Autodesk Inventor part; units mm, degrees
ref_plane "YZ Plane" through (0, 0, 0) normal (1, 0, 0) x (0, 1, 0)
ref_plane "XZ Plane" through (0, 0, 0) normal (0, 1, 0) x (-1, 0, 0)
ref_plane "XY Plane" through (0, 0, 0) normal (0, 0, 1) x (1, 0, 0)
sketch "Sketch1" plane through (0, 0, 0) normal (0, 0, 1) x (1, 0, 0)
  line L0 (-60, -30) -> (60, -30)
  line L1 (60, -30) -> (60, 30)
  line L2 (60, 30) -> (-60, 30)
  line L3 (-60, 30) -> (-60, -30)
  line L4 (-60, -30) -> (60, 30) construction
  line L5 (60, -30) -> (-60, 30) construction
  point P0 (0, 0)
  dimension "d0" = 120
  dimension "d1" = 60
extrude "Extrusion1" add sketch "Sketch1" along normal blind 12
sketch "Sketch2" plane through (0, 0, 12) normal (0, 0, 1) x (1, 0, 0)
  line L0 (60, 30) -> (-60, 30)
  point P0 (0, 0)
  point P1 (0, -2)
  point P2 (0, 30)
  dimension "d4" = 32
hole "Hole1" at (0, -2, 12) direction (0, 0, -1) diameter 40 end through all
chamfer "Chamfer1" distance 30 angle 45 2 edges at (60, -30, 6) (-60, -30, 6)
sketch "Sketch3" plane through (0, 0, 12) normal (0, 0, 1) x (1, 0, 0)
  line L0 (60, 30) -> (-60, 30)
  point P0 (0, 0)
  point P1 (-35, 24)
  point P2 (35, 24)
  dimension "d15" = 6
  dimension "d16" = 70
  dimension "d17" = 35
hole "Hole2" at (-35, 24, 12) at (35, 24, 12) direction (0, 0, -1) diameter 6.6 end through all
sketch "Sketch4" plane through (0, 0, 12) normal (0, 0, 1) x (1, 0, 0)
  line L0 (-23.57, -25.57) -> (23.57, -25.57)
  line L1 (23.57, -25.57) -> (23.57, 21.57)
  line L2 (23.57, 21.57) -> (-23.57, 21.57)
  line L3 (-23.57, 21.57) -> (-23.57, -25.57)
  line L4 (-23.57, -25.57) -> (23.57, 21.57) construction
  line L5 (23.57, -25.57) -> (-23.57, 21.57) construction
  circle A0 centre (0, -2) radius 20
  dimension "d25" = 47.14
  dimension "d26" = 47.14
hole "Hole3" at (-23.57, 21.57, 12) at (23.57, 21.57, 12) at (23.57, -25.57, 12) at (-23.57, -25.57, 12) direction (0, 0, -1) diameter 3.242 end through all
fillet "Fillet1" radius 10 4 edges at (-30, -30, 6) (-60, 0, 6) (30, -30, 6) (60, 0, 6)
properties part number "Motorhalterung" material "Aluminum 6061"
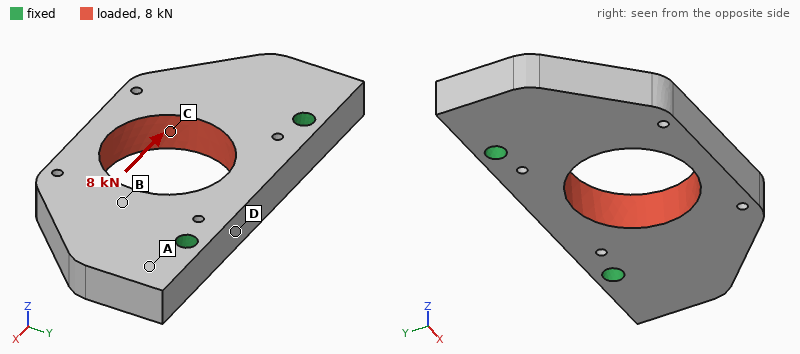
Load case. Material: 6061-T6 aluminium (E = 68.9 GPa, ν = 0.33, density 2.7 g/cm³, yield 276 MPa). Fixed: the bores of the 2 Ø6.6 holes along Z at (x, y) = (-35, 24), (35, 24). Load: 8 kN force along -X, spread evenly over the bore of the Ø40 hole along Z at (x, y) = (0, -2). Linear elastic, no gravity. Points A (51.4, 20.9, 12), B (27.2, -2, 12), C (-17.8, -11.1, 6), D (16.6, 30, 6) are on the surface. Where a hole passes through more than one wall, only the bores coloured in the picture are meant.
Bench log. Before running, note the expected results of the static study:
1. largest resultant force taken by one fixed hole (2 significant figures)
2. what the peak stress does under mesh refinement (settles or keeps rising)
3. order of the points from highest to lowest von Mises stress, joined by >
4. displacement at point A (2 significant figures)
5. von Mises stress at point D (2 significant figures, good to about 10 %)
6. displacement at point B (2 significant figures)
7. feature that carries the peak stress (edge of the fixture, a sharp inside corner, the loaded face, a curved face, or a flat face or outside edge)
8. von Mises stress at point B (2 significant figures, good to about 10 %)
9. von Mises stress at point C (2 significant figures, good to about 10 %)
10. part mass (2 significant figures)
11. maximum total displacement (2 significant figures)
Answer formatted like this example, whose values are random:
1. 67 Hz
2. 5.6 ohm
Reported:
1. 4.5 kN
2. keeps rising
3. D > C > B > A
4. 16 µm
5. 37 MPa
6. 26 µm
7. edge of the fixture
8. 17 MPa
9. 27 MPa
10. 160 g
11. 49 µm
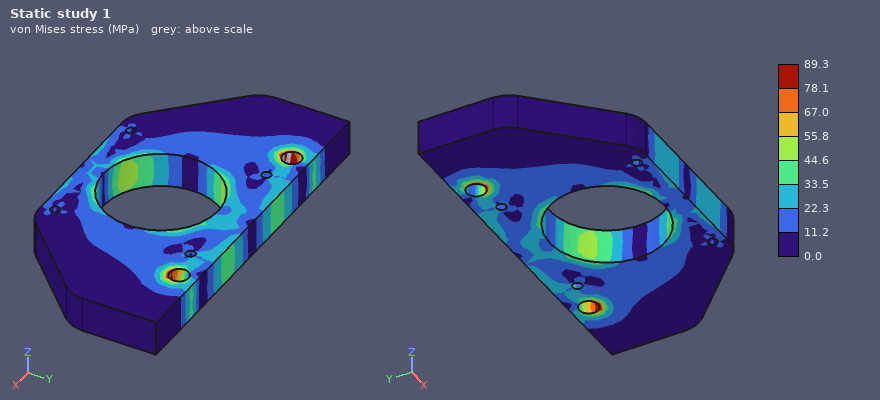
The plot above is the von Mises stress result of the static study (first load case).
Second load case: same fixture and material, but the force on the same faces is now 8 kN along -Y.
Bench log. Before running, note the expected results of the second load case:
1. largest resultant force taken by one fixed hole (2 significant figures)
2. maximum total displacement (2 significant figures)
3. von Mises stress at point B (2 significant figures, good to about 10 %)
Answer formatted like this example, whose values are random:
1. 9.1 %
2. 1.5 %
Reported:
1. 4.1 kN
2. 18 µm
3. 15 MPa
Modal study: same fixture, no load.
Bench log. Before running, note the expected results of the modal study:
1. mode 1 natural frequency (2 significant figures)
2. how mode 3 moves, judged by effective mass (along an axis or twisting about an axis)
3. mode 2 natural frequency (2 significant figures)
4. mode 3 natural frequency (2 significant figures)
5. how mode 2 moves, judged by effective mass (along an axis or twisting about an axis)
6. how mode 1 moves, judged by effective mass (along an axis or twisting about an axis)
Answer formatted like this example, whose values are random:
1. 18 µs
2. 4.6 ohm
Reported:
1. 3000 Hz
2. along X
3. 5100 Hz
4. 6500 Hz
5. twisting about Y
6. along Z
